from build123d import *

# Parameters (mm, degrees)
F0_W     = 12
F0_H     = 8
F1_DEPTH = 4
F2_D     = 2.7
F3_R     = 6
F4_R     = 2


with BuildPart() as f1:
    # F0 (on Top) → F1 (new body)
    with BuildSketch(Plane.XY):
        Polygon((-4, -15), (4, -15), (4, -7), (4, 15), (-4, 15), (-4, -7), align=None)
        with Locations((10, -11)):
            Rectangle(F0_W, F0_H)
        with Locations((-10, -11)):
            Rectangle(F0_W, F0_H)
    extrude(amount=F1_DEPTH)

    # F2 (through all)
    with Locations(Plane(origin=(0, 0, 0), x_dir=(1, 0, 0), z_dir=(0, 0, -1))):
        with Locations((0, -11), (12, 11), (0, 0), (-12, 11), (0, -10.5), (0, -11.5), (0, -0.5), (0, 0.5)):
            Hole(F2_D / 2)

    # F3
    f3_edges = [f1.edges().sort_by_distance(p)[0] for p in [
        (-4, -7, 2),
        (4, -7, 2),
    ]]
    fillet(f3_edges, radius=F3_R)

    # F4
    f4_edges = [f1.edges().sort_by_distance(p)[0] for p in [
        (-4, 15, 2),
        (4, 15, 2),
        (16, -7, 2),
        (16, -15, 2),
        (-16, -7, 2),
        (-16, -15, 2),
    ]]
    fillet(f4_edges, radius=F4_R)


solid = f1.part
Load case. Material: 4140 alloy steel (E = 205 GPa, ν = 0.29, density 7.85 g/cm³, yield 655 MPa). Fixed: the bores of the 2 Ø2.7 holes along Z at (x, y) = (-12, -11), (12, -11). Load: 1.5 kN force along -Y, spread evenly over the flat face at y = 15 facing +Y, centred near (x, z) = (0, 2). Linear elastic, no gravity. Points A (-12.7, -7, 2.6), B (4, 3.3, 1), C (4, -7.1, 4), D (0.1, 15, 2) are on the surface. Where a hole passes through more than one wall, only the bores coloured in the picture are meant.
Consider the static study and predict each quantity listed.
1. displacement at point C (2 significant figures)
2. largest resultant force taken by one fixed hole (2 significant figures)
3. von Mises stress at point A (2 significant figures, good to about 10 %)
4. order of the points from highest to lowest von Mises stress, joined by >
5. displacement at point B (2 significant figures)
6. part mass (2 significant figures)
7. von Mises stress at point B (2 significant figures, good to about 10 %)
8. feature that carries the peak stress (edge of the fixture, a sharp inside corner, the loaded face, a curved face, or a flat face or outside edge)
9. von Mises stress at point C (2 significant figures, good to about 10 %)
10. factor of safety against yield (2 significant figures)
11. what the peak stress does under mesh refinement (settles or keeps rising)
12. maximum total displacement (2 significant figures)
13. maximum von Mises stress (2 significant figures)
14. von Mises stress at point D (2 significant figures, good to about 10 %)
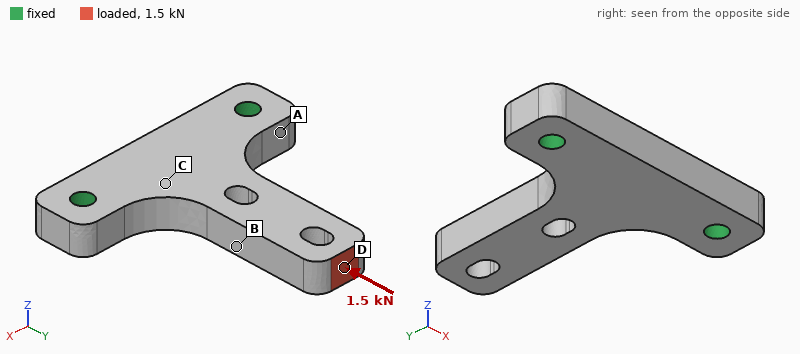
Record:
3.9 µm
810 N
16 MPa
D > B > C > A
6.5 µm
13 g
64 MPa
a curved face
34 MPa
2.6
settles
12 µm
250 MPa
120 MPa
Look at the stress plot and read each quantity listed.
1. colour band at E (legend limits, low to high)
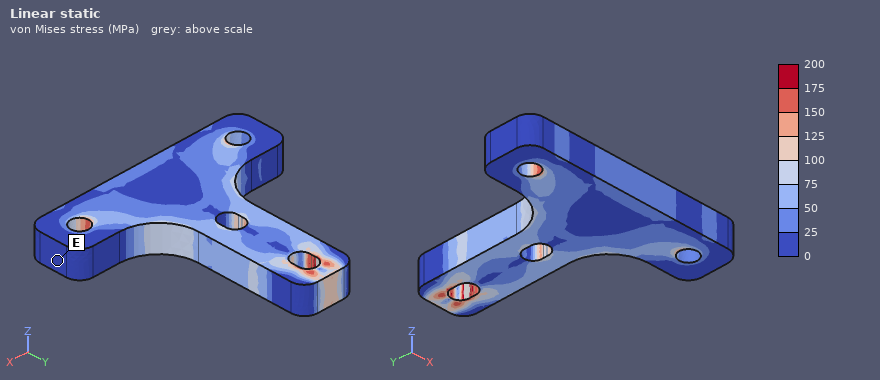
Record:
0 to 25 MPa
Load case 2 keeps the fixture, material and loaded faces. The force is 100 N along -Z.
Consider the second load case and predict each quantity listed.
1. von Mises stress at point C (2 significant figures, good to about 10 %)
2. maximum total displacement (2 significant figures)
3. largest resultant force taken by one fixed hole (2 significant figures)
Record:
70 MPa
78 µm
50 N
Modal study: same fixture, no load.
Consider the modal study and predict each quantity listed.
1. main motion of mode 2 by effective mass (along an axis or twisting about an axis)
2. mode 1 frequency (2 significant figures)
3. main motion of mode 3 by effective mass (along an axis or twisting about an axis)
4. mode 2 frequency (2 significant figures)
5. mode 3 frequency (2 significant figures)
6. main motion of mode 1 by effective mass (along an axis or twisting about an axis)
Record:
along X
4800 Hz
along Z
13 kHz
23 kHz
along Z
